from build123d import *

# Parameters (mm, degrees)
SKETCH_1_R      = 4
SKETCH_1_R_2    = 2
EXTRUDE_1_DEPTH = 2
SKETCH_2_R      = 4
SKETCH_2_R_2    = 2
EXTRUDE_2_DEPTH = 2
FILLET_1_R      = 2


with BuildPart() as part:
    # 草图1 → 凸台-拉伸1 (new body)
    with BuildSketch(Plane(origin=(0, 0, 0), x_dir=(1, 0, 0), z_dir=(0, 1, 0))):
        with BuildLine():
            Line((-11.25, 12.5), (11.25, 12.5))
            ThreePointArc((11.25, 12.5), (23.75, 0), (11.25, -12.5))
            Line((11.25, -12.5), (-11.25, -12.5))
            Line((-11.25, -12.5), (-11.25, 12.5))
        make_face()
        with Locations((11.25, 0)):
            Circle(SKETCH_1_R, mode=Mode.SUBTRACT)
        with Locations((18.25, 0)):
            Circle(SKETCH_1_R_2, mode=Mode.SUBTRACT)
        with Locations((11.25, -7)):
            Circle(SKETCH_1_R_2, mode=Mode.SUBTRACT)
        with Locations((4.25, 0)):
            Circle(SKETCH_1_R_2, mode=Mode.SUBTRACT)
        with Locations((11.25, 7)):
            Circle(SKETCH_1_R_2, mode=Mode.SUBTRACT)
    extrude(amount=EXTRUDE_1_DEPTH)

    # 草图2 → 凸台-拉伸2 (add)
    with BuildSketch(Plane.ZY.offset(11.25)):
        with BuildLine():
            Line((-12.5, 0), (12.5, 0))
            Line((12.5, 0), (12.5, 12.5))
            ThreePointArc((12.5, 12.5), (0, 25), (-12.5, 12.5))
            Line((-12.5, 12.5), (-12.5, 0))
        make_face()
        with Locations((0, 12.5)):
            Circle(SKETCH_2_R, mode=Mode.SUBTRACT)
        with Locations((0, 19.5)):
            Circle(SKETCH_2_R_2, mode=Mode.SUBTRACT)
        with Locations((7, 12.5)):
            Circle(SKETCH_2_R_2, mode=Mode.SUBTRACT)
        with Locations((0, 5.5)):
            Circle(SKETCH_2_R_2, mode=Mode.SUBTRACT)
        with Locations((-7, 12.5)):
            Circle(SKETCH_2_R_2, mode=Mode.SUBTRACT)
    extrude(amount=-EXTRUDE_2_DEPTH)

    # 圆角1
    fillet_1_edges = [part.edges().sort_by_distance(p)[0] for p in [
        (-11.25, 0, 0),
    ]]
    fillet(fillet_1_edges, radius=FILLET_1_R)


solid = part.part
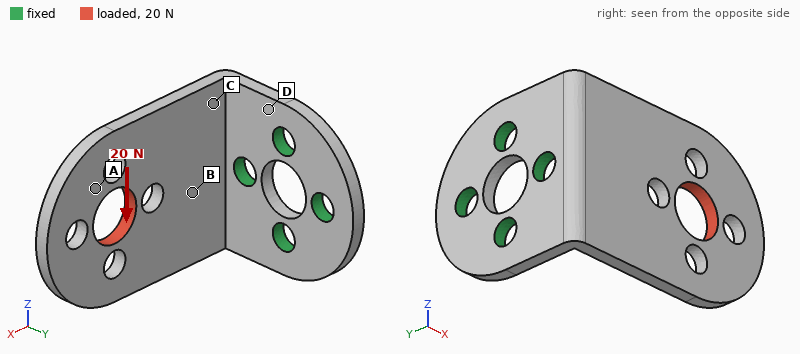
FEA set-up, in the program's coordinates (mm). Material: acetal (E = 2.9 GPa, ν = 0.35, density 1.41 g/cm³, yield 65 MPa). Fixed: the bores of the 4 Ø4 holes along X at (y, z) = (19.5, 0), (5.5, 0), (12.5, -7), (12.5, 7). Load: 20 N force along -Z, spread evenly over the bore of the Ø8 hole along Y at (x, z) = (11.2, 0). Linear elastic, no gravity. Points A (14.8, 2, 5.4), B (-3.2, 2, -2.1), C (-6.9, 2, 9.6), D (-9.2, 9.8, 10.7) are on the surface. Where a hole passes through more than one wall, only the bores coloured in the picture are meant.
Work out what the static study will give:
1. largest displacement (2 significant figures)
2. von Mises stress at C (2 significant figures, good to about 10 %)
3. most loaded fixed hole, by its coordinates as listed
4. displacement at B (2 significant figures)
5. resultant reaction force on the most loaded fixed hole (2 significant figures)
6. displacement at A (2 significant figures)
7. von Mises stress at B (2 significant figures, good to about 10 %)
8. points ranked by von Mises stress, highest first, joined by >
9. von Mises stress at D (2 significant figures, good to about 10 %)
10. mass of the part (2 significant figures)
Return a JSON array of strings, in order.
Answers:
["0.54 mm", "6.2 MPa", "(5.5, 0)", "0.12 mm", "17 N", "0.42 mm", "3.8 MPa", "D > C > B > A", "8.6 MPa", "3.1 g"]
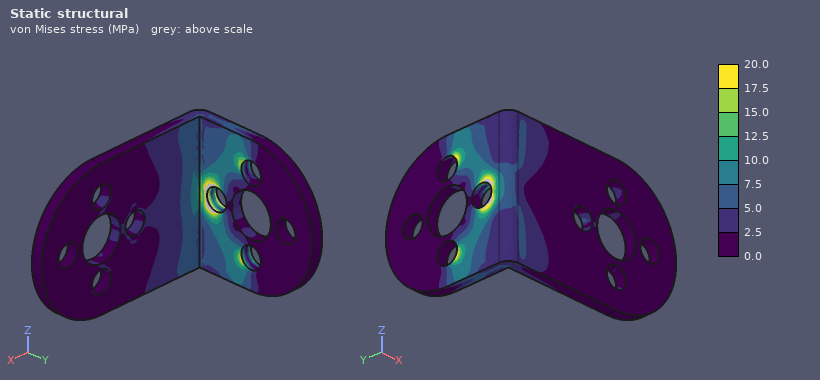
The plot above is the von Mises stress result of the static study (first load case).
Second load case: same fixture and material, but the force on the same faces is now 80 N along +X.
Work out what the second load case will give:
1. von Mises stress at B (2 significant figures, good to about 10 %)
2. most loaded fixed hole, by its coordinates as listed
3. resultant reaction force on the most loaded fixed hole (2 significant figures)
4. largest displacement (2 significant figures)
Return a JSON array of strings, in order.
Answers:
["3.0 MPa", "(5.5, 0)", "85 N", "0.49 mm"]
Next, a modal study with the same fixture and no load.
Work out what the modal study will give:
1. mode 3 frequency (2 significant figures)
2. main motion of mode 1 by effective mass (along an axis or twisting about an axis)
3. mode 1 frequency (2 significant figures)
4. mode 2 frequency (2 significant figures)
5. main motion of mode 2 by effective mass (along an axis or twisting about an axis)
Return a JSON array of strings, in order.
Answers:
["1400 Hz", "along Y", "430 Hz", "950 Hz", "along Z"]
